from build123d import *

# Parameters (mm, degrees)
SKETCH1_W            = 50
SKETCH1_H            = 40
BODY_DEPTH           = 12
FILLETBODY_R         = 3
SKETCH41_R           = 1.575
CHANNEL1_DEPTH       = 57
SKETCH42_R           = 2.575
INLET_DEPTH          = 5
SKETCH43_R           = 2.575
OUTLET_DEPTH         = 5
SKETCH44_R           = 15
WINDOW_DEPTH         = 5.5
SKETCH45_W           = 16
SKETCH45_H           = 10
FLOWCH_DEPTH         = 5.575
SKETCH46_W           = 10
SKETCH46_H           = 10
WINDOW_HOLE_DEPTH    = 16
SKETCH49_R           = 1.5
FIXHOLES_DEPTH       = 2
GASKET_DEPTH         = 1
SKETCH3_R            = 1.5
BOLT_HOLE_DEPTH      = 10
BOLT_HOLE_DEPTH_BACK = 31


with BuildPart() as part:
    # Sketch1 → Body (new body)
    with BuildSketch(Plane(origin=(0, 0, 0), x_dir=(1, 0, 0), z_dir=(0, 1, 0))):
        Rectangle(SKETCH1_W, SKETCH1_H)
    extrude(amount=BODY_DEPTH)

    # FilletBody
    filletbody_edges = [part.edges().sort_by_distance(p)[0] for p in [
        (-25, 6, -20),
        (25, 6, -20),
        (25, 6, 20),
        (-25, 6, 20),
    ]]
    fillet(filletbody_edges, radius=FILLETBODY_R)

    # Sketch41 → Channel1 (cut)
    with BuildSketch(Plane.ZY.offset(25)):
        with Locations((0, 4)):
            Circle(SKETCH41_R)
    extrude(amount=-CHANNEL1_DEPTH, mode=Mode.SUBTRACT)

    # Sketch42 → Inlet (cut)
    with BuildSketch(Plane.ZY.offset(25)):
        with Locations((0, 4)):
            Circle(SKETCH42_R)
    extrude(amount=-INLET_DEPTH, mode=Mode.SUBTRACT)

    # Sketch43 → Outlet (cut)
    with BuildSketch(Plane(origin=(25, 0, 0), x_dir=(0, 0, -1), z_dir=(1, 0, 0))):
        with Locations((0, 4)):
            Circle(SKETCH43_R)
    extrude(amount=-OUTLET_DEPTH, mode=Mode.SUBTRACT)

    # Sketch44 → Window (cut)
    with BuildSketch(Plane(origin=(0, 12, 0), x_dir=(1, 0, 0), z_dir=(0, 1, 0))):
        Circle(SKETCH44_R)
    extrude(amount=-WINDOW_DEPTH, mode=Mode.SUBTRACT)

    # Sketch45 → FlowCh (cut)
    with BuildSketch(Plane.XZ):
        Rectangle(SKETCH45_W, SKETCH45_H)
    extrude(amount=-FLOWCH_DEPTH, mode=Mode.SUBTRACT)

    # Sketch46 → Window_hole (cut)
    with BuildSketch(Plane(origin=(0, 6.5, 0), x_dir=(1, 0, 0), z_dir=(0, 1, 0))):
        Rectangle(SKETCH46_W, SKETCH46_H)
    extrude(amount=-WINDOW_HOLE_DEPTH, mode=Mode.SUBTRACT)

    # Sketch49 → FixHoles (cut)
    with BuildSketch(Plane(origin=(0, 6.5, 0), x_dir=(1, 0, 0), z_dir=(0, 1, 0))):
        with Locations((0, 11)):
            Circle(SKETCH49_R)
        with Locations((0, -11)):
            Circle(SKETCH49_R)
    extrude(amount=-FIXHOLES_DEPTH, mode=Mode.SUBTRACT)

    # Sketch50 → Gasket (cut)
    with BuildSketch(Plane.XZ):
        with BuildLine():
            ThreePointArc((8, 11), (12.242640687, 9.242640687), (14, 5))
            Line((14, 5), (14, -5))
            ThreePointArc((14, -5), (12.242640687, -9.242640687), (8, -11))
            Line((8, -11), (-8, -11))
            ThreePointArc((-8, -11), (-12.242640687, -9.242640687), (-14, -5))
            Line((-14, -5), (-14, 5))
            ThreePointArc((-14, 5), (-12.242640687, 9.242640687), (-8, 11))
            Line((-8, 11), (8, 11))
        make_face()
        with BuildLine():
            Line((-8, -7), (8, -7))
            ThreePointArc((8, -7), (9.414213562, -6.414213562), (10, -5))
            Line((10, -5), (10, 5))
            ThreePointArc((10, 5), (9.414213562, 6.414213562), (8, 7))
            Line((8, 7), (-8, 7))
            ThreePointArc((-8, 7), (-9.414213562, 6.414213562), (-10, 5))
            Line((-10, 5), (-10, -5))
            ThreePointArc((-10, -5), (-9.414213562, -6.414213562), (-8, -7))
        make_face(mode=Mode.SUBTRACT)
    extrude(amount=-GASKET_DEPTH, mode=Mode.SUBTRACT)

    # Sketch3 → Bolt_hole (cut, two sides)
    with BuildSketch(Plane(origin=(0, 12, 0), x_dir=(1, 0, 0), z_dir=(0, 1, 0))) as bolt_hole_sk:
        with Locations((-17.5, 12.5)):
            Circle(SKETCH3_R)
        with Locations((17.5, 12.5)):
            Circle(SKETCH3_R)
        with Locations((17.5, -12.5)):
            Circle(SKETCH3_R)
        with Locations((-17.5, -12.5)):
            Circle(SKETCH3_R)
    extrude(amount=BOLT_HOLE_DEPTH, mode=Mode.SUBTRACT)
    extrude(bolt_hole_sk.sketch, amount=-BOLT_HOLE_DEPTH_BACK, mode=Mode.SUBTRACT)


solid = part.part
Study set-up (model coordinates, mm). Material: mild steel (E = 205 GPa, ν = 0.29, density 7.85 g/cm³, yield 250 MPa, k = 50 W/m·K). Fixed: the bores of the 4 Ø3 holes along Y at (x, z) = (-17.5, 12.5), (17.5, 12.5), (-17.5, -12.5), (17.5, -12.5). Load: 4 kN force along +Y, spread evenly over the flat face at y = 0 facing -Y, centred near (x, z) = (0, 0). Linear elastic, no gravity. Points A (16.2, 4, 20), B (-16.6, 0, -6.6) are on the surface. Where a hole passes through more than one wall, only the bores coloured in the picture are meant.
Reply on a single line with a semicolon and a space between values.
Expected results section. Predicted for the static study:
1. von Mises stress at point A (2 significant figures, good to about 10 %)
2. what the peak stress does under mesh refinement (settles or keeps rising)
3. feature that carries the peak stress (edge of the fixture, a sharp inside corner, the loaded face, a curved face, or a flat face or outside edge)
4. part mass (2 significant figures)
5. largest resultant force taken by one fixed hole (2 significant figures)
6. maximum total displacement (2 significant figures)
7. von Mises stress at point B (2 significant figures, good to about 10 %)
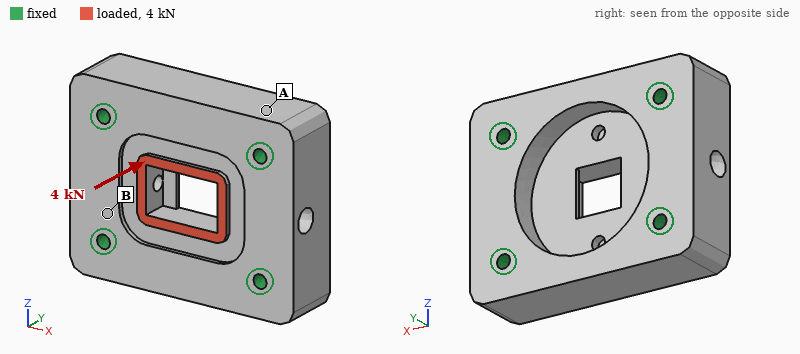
7.9 MPa; keeps rising; edge of the fixture; 140 g; 1.0 kN; 8.5 µm; 20 MPa
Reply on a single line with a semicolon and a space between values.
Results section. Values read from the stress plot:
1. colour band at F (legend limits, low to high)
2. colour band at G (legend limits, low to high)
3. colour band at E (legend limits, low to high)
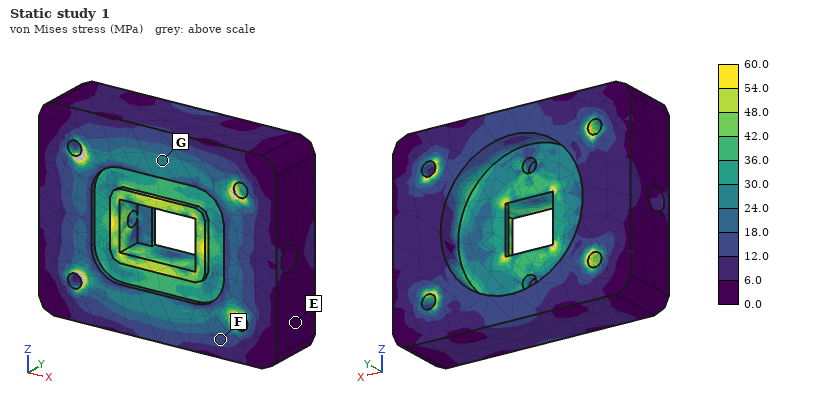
12.0 to 18.0 MPa; 24.0 to 30.0 MPa; 0.0 to 6.0 MPa
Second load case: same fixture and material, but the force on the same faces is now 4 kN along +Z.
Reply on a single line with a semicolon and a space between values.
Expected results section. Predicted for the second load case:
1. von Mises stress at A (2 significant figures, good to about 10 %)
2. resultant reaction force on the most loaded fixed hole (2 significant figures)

7.9 MPa; 1.1 kN
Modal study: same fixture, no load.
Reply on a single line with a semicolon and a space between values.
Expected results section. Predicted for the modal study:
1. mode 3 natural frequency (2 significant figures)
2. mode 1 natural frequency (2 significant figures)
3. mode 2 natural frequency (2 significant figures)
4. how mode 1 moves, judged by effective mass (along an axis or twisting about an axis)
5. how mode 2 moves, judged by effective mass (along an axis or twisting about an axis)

35 kHz; 30 kHz; 32 kHz; along Y; twisting about X
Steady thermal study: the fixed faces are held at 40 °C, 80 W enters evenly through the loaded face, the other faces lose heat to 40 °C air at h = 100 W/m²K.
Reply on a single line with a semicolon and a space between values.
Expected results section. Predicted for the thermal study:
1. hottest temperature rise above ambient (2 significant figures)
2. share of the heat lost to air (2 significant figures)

77 K; 12 %
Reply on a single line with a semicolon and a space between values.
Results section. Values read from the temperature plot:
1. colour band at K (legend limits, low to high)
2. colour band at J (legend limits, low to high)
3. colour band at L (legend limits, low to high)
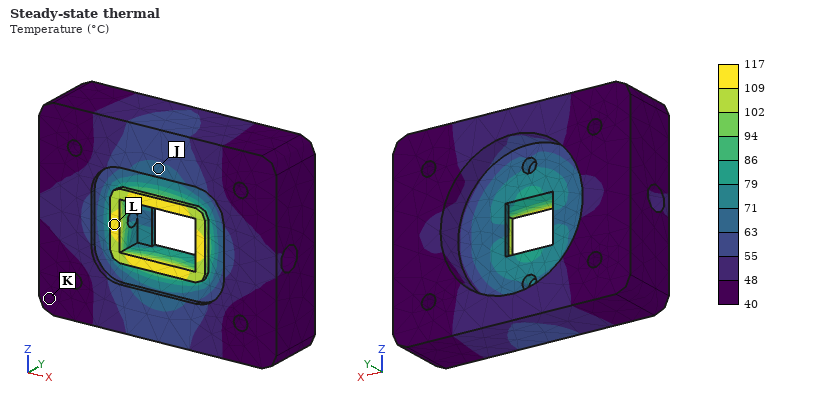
40 to 48 °C; 63 to 71 °C; 109 to 117 °C
